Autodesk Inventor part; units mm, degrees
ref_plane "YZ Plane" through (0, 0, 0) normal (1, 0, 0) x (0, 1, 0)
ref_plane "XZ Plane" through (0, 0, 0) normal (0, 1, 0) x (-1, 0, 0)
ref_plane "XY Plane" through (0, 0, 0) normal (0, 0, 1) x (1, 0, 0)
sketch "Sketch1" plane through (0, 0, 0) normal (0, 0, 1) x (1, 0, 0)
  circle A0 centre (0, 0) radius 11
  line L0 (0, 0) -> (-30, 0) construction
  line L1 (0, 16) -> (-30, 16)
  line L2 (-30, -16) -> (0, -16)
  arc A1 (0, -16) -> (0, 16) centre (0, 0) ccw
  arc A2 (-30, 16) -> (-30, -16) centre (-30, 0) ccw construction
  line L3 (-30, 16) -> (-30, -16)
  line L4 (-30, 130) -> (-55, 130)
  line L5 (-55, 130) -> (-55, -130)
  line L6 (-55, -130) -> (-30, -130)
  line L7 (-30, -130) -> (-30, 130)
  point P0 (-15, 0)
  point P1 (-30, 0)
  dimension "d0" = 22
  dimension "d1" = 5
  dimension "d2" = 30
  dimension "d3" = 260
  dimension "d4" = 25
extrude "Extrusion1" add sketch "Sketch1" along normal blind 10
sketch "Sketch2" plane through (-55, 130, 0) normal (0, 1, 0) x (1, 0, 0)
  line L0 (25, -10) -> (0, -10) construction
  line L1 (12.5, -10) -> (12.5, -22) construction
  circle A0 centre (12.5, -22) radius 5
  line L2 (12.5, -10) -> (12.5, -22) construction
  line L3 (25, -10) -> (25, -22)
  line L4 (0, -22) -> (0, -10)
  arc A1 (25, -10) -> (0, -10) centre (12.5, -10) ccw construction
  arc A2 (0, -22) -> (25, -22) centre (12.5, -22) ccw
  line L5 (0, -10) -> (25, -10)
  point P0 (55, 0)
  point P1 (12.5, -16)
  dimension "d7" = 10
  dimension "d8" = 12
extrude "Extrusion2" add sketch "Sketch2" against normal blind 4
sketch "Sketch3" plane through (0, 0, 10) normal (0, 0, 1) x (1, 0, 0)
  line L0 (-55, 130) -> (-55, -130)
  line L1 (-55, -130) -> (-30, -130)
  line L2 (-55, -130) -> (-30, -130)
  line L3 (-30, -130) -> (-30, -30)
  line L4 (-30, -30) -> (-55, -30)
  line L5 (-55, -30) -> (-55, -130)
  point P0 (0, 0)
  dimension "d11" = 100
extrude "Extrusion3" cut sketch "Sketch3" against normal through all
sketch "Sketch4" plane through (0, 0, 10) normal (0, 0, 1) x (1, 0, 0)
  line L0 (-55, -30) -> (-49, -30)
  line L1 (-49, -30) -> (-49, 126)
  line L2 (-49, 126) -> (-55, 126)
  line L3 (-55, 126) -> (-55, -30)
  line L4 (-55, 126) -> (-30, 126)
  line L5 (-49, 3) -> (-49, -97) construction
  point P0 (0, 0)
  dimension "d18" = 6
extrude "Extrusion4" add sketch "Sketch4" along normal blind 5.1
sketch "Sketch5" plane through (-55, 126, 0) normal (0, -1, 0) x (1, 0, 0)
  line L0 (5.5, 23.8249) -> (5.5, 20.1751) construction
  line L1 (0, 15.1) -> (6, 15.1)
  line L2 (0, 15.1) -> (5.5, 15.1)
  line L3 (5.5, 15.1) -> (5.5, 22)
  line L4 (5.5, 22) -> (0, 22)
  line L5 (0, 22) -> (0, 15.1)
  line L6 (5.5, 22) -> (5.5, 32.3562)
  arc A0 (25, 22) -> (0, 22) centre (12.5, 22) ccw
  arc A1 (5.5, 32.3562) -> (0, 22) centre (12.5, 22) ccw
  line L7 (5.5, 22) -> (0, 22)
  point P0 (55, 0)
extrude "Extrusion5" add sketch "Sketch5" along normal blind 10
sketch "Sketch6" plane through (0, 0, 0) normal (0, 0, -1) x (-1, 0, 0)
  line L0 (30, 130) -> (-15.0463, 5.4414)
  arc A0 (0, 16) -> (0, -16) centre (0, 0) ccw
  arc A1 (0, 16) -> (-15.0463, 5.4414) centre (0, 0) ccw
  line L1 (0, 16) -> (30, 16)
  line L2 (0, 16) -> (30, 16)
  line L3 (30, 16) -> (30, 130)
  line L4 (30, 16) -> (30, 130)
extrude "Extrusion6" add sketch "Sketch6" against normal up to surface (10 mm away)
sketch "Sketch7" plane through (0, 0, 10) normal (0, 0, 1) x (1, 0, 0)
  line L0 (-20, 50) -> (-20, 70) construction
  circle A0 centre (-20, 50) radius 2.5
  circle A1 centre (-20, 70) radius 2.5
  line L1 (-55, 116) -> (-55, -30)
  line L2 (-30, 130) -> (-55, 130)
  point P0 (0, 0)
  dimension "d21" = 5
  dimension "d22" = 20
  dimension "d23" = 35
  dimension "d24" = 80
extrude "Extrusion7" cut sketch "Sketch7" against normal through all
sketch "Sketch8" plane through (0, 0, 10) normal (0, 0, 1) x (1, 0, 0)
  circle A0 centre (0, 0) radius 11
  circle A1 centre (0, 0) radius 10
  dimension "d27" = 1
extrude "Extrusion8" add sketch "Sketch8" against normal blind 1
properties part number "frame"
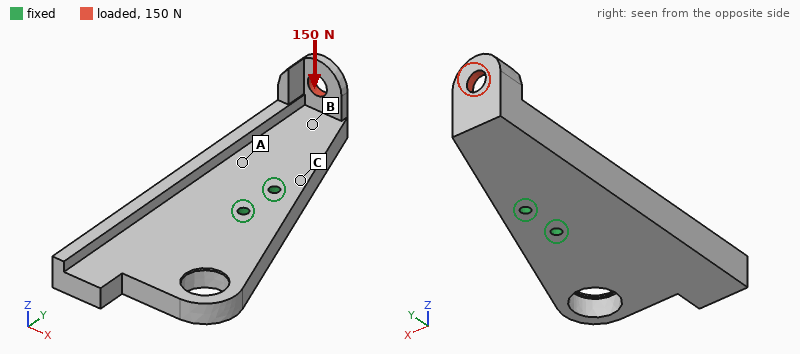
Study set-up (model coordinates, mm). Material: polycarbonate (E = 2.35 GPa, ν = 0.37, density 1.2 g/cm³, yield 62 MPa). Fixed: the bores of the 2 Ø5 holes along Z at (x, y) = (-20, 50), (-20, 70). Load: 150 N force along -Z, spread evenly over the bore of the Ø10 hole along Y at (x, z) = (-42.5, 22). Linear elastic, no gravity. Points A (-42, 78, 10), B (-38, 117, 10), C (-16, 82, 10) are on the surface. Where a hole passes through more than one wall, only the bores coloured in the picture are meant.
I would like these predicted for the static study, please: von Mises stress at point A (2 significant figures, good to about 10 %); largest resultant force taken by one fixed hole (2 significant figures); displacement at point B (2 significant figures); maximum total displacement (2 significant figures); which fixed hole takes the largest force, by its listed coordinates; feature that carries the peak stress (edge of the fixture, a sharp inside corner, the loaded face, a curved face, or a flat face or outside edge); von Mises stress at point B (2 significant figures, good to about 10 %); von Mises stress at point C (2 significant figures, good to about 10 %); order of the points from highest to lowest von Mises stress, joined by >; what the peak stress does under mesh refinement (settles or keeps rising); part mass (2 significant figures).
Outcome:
5.6 MPa
350 N
1.1 mm
1.8 mm
(-20, 70)
edge of the fixture
2.5 MPa
11 MPa
C > A > B
keeps rising
97 g
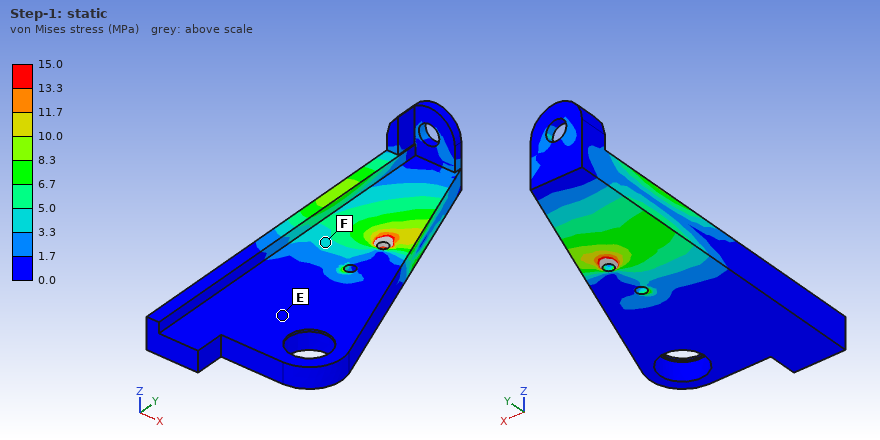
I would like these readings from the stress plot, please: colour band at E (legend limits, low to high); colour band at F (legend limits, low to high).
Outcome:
0.0 to 1.7 MPa
3.3 to 5.0 MPa
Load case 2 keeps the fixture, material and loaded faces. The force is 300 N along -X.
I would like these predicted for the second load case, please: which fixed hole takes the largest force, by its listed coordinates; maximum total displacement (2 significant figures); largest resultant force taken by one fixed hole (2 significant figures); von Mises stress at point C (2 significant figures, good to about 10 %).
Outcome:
(-20, 70)
1.8 mm
1.0 kN
7.5 MPa
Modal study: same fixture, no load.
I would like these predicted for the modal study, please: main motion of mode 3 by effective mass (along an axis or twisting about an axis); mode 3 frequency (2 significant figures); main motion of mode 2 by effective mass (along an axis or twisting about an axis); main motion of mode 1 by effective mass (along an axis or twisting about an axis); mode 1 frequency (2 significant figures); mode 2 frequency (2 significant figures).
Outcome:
twisting about Y
760 Hz
along Z
along Z
370 Hz
500 Hz
